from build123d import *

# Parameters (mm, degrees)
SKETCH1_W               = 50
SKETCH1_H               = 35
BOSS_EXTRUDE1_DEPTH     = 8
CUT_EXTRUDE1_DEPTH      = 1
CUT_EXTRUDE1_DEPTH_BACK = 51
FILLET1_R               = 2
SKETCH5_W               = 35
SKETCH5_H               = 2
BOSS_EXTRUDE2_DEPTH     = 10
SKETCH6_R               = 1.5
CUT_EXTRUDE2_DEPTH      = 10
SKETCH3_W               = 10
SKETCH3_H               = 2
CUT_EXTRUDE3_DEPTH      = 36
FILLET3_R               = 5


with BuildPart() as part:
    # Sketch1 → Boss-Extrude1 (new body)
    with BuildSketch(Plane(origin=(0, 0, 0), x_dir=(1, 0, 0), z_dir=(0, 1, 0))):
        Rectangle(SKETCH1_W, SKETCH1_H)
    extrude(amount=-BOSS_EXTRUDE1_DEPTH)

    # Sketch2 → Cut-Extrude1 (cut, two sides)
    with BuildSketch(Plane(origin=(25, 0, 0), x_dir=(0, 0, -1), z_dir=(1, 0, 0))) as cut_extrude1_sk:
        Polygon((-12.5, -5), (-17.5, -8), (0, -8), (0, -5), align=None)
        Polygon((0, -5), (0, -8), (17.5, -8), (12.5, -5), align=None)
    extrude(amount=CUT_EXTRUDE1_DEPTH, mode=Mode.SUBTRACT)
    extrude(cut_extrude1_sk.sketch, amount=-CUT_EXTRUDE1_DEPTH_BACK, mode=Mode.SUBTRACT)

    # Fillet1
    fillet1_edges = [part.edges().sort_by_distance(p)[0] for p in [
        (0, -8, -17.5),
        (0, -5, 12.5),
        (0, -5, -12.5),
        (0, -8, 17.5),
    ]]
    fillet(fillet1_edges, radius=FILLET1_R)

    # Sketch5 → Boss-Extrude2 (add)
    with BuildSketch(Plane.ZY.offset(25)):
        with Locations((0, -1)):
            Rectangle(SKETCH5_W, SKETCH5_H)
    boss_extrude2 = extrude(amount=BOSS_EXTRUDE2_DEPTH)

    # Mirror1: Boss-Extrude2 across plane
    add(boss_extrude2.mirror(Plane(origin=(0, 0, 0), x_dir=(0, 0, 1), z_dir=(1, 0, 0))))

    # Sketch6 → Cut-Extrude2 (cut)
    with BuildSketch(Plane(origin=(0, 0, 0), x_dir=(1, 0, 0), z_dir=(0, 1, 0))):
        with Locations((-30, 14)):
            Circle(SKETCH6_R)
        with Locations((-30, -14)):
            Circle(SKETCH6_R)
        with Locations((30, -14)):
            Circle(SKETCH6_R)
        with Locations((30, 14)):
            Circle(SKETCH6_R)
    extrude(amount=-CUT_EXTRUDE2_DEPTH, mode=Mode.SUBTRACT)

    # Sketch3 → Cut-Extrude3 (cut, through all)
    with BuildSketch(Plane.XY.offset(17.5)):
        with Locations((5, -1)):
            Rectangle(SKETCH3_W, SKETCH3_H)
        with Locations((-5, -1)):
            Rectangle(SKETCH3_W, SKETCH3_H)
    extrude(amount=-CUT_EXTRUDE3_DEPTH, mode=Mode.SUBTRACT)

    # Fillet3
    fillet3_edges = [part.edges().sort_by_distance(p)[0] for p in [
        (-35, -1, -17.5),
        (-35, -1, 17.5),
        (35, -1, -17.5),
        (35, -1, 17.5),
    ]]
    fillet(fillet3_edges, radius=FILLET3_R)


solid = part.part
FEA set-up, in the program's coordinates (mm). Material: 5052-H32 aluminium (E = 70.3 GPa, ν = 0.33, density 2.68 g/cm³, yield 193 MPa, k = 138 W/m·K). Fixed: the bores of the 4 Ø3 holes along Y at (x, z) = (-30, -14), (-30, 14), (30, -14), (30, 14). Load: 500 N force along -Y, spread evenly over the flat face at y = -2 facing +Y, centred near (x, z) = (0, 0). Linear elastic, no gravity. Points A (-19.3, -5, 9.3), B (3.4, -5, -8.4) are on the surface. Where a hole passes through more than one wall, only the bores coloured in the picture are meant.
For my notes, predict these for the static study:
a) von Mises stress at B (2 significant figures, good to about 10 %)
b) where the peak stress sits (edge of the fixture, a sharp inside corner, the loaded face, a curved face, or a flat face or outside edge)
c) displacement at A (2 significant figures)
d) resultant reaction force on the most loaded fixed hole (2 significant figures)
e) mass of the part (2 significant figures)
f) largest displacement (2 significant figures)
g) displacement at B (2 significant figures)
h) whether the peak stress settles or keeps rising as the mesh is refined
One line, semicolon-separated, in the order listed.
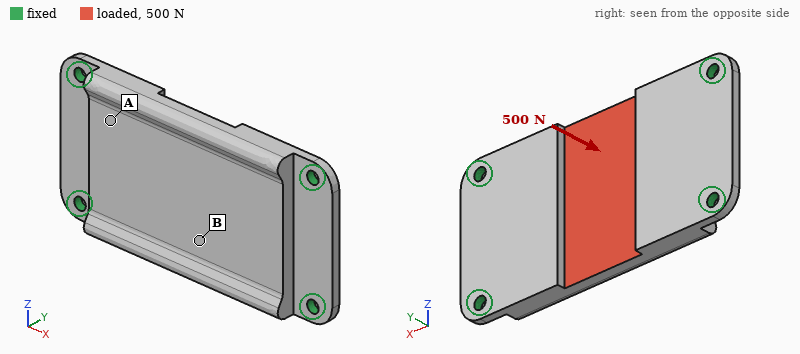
31 MPa; edge of the fixture; 22 µm; 570 N; 24 g; 54 µm; 51 µm; keeps rising
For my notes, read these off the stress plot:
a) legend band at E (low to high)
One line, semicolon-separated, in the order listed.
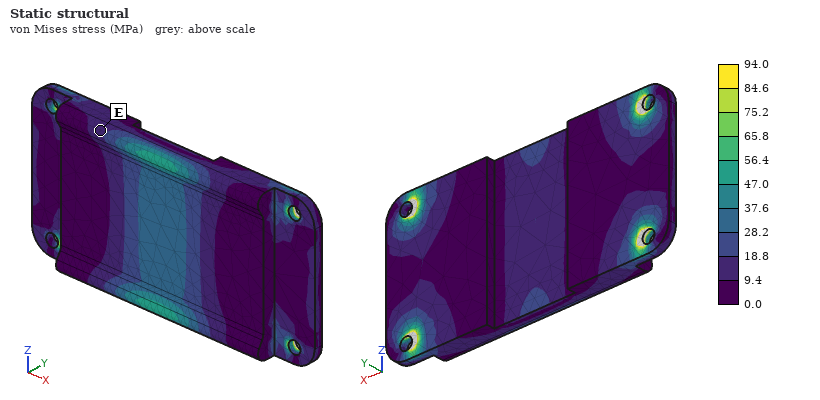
9.4 to 18.8 MPa
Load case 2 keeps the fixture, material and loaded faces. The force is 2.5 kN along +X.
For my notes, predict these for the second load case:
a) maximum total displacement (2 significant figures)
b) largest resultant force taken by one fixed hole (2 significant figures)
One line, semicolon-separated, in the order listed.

13 µm; 640 N
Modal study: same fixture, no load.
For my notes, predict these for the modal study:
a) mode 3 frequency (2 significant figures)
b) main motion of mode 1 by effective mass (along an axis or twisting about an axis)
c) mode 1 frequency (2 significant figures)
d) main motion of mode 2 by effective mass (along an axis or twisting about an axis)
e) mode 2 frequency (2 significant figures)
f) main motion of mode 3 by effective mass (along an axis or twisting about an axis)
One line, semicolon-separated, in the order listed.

11 kHz; along Y; 4900 Hz; twisting about X; 8200 Hz; twisting about Z
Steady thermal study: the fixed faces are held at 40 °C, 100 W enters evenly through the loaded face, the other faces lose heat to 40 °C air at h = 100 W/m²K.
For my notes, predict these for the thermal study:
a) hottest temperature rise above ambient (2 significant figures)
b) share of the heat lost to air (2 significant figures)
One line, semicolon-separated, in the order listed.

80 K; 23 %
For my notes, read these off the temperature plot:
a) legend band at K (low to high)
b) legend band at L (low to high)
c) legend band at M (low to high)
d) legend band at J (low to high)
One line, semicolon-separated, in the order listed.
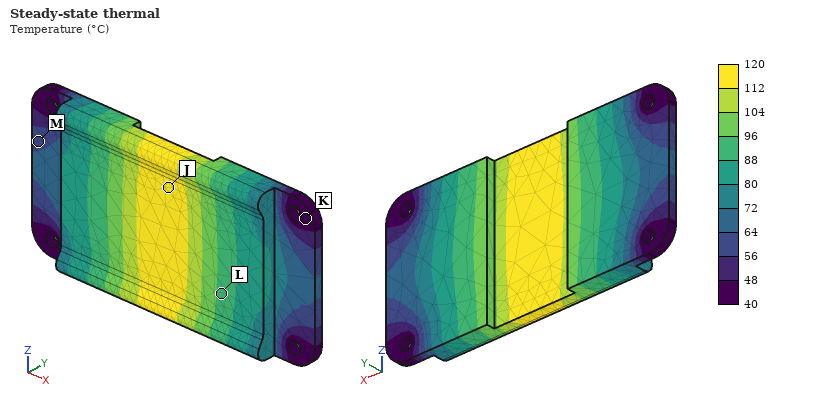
40 to 48 °C; 88 to 96 °C; 56 to 64 °C; 112 to 120 °C
